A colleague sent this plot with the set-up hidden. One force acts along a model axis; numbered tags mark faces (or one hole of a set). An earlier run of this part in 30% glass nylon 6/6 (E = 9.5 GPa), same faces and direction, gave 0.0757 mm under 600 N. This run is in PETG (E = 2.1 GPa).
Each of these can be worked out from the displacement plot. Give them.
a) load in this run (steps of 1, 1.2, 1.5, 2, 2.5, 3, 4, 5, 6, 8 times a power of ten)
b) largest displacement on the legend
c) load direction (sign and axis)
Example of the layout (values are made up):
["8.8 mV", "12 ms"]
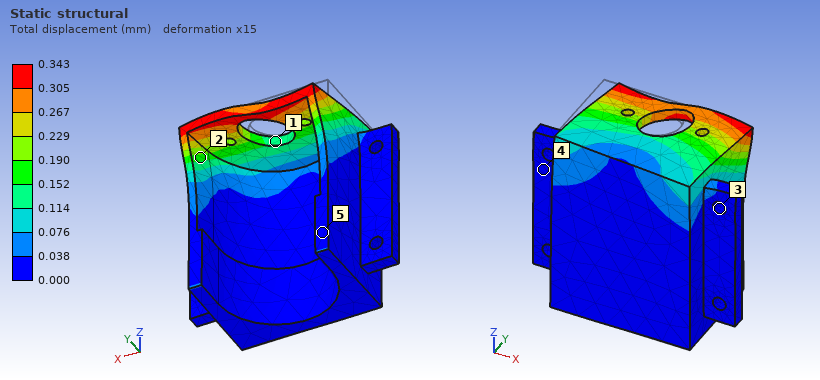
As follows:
["600 N", "0.343 mm", "+X"]
